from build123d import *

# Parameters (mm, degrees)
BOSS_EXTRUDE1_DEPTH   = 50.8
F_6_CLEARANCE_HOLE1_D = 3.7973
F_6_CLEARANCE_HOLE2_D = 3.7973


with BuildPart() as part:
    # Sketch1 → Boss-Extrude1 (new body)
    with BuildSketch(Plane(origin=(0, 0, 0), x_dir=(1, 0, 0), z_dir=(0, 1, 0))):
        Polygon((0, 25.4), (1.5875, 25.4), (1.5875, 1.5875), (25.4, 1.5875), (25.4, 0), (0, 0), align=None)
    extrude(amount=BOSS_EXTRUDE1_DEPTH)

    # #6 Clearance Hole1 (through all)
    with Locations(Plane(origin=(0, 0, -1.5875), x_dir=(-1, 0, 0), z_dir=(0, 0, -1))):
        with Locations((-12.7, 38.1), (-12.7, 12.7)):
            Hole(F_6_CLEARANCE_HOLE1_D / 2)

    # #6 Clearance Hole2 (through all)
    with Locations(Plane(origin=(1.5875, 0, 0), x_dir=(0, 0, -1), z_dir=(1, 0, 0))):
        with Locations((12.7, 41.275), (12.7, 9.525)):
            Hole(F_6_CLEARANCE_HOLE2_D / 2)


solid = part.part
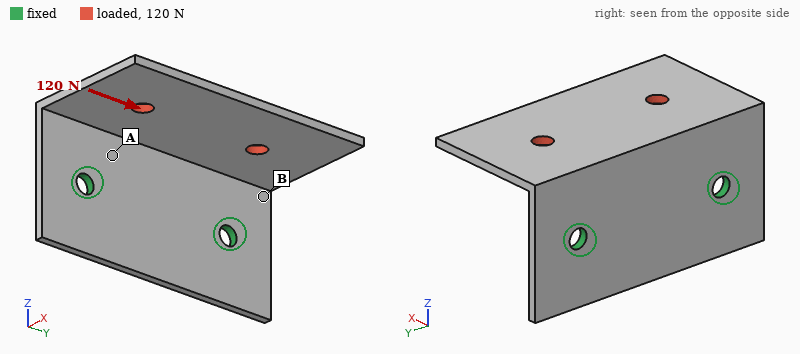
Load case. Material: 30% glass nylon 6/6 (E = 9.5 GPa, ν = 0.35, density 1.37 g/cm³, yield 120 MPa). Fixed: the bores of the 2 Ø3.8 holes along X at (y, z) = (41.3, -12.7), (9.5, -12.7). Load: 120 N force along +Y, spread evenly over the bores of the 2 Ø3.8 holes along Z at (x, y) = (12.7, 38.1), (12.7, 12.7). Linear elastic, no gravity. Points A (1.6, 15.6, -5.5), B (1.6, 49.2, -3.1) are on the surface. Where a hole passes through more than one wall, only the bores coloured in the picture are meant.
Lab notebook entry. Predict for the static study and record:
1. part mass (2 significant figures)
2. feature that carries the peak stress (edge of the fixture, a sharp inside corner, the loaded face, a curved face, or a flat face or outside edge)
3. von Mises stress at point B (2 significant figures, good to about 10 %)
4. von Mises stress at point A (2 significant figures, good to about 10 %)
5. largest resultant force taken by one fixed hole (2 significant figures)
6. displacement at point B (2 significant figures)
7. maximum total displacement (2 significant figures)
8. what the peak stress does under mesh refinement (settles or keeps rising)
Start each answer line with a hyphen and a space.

- 5.3 g
- edge of the fixture
- 8.4 MPa
- 18 MPa
- 83 N
- 0.22 mm
- 0.55 mm
- keeps rising
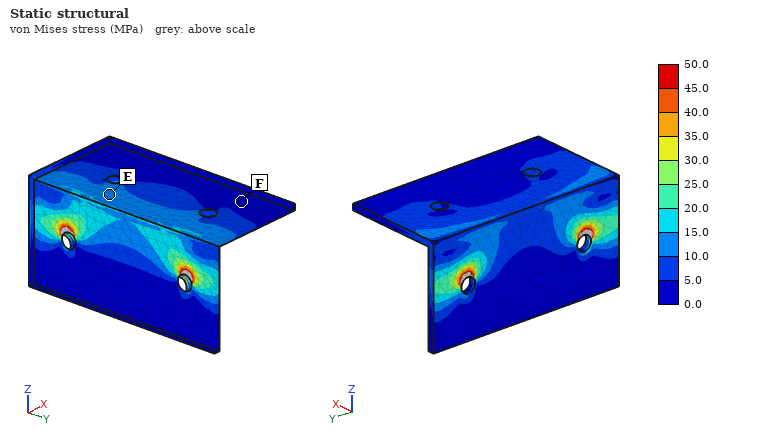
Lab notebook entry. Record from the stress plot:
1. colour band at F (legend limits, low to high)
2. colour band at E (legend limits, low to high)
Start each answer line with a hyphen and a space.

- 0.0 to 5.0 MPa
- 10.0 to 15.0 MPa
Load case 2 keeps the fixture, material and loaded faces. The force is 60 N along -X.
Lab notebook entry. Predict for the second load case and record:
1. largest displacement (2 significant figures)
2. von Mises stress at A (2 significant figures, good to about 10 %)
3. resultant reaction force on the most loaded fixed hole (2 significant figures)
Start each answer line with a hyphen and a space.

- 0.68 mm
- 13 MPa
- 30 N
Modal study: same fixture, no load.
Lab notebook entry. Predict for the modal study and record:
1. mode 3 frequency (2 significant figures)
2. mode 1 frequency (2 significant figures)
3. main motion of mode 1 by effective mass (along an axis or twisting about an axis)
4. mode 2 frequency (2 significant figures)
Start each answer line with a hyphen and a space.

- 2000 Hz
- 650 Hz
- along Z
- 1200 Hz
